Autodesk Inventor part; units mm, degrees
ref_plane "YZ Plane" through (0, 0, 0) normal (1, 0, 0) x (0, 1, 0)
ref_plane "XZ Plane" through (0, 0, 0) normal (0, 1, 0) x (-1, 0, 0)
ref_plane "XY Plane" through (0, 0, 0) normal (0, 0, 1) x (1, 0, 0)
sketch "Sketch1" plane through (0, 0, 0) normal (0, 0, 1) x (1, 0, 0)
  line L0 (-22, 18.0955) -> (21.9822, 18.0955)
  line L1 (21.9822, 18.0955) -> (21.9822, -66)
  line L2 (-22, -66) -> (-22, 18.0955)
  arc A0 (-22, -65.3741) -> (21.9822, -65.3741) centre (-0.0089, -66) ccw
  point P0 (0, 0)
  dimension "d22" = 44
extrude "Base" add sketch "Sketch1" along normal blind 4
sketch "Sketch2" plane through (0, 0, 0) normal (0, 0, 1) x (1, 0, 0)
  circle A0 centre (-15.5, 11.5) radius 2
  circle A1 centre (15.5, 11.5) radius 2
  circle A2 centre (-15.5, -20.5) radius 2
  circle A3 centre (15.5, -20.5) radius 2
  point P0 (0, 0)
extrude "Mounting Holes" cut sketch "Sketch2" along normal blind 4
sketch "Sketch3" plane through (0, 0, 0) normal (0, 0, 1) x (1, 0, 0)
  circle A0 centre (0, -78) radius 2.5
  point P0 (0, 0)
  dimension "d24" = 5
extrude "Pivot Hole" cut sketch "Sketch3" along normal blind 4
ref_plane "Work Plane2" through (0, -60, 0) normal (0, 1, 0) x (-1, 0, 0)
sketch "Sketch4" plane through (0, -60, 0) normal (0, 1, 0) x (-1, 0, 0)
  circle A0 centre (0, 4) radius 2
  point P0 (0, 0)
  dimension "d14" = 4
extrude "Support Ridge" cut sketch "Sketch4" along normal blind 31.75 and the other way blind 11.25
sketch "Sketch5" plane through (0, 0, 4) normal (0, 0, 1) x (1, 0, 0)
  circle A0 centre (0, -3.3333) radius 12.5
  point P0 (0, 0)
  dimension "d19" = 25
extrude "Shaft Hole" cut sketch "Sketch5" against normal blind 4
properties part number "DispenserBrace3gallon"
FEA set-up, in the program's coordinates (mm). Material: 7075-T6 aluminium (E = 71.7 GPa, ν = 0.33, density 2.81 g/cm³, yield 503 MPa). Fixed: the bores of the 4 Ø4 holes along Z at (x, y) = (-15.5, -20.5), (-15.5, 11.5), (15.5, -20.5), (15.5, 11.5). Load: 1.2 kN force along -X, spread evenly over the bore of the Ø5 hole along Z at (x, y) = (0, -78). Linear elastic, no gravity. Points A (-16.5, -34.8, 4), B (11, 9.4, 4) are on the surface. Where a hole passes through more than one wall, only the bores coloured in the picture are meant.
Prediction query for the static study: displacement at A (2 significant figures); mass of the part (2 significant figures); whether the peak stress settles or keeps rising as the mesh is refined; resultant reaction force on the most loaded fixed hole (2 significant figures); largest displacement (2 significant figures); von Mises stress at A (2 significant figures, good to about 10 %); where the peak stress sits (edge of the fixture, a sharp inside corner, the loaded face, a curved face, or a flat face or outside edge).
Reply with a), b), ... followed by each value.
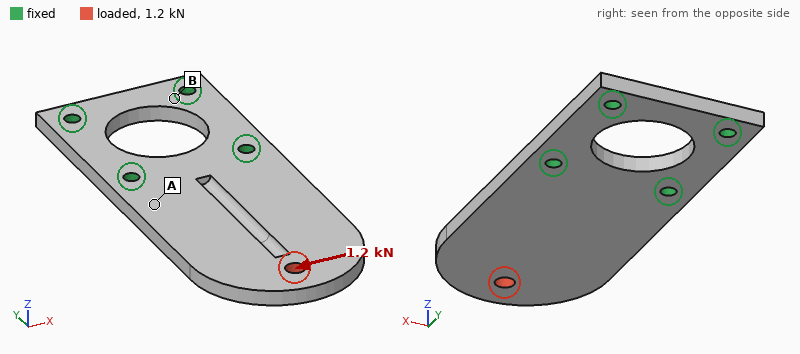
a) 12 µm
b) 43 g
c) keeps rising
d) 2.1 kN
e) 71 µm
f) 31 MPa
g) edge of the fixture
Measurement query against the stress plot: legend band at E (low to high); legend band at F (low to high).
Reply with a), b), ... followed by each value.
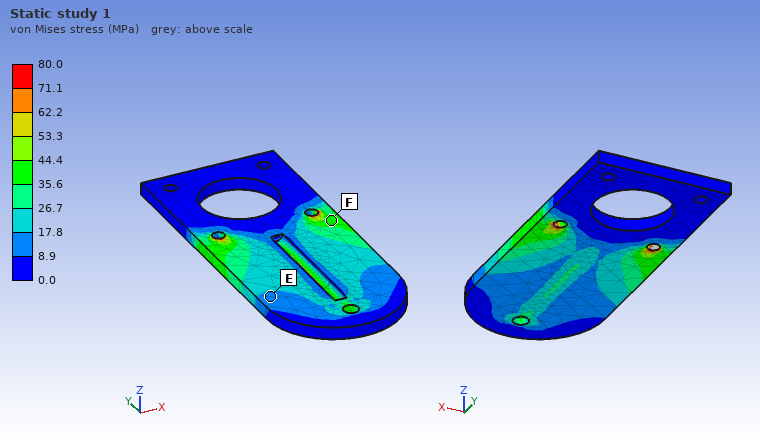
a) 8.9 to 17.8 MPa
b) 35.6 to 44.4 MPa
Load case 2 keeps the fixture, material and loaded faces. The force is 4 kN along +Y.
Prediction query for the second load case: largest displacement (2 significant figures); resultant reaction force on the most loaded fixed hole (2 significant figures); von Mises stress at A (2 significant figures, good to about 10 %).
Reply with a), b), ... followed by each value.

a) 37 µm
b) 1.9 kN
c) 29 MPa
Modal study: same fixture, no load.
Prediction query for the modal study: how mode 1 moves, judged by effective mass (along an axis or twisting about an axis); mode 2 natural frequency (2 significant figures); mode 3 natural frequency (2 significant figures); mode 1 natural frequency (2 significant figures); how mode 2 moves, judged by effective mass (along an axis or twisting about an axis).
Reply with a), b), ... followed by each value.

a) along Z
b) 2800 Hz
c) 4700 Hz
d) 800 Hz
e) twisting about Y
